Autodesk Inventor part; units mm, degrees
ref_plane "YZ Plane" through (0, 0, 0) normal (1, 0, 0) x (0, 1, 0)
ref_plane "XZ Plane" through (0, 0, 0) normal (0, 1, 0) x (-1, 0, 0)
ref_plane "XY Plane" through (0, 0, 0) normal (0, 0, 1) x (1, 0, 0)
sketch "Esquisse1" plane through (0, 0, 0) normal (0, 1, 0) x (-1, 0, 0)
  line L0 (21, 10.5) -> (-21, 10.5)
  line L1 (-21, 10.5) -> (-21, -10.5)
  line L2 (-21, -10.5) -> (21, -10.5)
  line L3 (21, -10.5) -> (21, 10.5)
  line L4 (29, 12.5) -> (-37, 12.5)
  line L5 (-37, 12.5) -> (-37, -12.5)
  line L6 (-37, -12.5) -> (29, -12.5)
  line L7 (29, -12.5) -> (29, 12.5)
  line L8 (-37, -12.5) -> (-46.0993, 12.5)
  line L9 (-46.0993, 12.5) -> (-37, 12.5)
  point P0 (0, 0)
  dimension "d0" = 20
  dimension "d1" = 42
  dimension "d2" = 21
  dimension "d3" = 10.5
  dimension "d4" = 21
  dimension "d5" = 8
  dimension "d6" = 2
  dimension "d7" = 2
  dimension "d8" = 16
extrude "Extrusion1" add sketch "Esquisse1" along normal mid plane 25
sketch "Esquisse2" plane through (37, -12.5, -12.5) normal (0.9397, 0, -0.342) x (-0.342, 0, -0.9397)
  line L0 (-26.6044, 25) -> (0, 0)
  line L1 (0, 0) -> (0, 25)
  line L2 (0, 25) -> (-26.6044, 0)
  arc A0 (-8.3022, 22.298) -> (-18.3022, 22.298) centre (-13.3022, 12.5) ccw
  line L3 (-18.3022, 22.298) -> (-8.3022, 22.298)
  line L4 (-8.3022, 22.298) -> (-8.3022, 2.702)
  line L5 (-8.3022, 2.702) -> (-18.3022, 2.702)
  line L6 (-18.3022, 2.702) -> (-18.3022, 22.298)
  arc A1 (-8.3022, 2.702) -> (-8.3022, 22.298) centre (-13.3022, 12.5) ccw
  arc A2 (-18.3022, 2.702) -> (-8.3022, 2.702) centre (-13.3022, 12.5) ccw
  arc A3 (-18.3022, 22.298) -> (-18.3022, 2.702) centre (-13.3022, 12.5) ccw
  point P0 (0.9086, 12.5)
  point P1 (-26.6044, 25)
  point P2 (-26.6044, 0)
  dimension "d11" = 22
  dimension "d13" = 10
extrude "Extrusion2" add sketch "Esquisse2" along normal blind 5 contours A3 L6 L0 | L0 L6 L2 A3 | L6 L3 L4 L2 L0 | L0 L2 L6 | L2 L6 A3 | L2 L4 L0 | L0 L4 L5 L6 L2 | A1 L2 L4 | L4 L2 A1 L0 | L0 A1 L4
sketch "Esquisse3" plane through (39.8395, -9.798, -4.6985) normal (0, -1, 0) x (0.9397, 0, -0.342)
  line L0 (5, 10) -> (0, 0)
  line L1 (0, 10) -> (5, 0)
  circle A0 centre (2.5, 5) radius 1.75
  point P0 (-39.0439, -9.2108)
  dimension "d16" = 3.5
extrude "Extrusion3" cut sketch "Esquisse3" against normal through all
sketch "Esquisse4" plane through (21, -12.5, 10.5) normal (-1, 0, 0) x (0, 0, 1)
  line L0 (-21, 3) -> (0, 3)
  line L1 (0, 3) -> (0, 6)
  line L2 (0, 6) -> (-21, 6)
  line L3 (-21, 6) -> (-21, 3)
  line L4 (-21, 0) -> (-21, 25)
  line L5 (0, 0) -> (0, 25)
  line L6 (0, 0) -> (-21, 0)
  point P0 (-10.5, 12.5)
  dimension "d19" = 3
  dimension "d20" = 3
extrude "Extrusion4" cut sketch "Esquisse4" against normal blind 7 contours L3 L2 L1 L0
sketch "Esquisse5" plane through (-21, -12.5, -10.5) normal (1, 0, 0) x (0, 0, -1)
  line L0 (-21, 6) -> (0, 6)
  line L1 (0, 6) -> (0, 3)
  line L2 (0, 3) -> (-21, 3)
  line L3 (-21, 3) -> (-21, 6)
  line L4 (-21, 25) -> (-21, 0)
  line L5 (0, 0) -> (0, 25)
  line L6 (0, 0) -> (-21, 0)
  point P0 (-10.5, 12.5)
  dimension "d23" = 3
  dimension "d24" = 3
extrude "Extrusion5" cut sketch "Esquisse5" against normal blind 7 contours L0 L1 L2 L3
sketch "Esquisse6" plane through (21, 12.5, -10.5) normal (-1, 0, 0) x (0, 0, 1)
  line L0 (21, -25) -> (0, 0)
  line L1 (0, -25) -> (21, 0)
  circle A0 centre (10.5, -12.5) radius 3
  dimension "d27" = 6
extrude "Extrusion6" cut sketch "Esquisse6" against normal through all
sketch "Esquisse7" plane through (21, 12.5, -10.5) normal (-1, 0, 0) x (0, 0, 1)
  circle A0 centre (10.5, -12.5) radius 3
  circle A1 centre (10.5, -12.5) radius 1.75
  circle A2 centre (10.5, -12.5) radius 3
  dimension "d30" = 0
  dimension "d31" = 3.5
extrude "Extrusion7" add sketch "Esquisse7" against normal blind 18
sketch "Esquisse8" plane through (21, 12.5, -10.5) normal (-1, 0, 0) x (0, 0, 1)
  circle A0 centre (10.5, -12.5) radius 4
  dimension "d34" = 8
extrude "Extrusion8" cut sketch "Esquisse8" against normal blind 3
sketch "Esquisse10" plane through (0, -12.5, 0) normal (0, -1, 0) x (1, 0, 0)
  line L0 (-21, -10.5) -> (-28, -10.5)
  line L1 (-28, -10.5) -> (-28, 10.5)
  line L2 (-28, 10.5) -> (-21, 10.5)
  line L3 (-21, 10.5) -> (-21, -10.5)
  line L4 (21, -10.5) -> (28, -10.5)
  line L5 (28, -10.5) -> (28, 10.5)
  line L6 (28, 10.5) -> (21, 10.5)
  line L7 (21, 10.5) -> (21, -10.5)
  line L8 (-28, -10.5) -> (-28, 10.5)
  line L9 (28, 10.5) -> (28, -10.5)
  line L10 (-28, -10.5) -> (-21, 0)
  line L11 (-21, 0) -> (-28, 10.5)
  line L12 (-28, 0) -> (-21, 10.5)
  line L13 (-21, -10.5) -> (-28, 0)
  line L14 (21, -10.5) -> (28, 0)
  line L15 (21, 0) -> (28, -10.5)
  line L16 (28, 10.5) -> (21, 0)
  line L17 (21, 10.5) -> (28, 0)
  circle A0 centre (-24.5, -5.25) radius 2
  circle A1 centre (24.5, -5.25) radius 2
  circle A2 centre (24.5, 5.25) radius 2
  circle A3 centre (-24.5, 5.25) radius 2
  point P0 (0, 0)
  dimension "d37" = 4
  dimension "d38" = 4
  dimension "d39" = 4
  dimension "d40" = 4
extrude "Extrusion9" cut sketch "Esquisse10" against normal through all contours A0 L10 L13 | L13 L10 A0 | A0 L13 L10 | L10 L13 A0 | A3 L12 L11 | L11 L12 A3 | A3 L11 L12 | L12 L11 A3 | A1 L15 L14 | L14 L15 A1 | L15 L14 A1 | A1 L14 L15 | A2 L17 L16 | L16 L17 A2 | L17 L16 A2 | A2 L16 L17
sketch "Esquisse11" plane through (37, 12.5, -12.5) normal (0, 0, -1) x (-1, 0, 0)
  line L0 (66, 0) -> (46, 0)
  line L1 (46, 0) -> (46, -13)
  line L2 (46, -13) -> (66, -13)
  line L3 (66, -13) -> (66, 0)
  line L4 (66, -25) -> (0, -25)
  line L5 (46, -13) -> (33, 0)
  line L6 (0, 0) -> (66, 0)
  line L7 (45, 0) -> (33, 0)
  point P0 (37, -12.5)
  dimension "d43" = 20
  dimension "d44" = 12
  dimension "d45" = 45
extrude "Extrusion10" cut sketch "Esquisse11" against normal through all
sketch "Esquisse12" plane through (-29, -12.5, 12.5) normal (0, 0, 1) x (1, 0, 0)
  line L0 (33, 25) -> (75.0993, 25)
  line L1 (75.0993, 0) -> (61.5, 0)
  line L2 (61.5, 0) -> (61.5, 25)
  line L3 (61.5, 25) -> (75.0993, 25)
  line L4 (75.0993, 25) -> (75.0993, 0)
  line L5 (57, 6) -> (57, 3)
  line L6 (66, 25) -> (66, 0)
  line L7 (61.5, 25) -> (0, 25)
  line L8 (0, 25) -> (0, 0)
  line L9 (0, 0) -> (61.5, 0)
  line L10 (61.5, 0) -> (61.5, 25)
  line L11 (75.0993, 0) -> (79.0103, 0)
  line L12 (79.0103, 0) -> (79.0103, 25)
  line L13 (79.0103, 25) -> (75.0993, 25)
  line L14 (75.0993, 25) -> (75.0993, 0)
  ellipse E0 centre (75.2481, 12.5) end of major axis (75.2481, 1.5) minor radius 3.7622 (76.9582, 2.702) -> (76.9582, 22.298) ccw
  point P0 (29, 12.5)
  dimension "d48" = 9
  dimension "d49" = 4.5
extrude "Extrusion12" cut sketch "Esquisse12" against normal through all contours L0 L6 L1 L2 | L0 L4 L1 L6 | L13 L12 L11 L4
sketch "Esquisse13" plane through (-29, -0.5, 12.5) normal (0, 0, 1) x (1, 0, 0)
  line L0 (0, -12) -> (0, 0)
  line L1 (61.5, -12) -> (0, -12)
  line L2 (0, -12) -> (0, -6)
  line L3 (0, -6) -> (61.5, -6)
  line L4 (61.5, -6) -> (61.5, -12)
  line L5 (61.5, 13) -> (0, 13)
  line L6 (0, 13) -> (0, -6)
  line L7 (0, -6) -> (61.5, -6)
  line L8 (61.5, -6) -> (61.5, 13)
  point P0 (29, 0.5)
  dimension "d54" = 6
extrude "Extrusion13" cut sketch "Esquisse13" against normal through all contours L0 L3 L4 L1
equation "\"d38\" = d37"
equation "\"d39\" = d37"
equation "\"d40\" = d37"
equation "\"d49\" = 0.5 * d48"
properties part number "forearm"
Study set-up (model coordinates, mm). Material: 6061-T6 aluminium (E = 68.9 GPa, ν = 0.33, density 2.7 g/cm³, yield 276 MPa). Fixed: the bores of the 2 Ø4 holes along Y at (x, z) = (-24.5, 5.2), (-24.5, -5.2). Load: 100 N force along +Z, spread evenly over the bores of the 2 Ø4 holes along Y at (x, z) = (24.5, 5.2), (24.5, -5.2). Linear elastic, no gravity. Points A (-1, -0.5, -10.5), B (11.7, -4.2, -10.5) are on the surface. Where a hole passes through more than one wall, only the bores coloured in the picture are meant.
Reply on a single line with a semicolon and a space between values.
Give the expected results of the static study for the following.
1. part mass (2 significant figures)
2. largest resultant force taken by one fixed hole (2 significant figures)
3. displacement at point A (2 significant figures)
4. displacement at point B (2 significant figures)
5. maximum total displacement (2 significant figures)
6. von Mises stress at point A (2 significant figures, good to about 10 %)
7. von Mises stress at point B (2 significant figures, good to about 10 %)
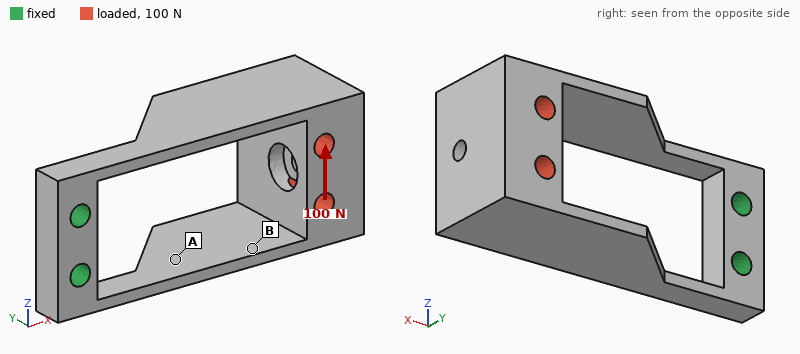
22 g; 200 N; 0.39 mm; 0.63 mm; 0.73 mm; 39 MPa; 78 MPa
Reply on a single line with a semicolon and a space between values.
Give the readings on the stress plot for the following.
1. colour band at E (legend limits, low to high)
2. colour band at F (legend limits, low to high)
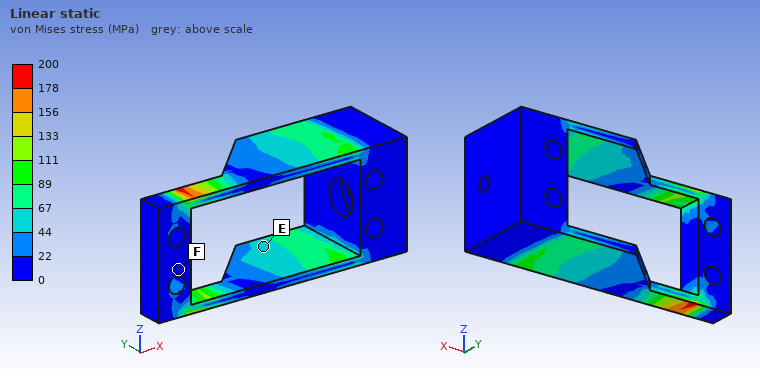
44 to 67 MPa; 0 to 22 MPa
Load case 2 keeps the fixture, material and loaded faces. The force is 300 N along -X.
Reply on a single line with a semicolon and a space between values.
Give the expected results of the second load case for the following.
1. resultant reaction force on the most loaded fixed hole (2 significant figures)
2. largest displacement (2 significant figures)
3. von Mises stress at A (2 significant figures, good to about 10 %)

150 N; 0.38 mm; 13 MPa
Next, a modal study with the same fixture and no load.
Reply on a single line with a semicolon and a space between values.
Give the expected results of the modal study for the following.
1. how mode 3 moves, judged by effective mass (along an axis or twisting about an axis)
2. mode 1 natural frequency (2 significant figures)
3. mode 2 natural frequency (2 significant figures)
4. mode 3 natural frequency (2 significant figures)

twisting about X; 460 Hz; 480 Hz; 2300 Hz
